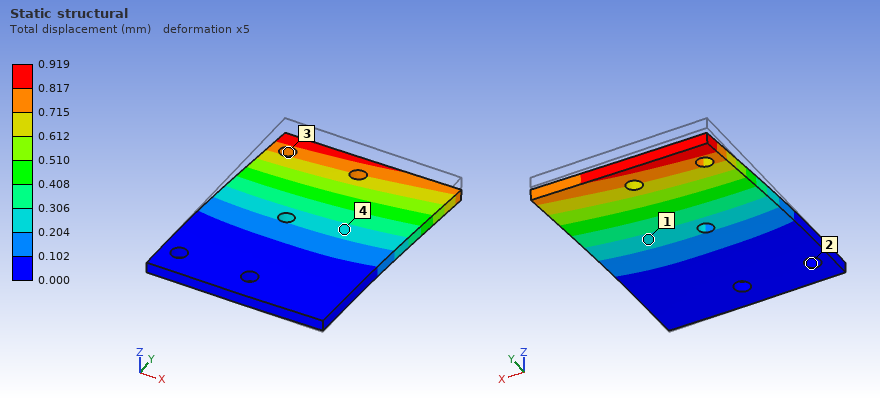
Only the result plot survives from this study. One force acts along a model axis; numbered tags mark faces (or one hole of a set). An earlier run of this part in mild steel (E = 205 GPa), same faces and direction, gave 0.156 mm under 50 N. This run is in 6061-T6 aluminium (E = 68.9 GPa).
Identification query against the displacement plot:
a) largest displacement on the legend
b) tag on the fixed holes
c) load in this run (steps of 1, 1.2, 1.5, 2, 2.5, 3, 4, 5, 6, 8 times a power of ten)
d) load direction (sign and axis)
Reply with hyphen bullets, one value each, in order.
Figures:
- 0.919 mm
- 2
- 100 N
- -Z
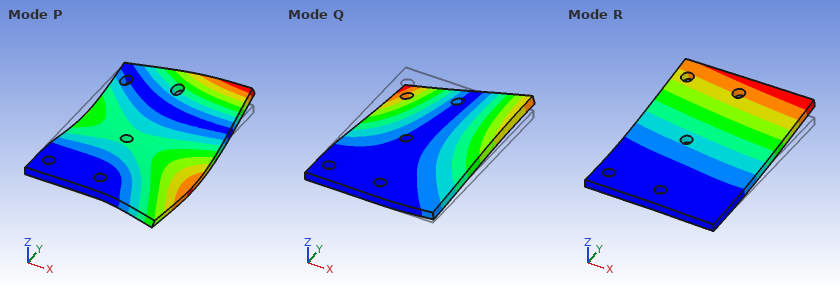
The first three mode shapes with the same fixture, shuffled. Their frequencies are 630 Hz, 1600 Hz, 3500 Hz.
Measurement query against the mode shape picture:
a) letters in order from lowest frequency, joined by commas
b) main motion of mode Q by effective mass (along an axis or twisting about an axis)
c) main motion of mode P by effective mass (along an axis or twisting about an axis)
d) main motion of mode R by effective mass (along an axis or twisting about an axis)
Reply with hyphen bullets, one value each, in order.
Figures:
- R, Q, P
- twisting about Y
- along Z
- along Z
